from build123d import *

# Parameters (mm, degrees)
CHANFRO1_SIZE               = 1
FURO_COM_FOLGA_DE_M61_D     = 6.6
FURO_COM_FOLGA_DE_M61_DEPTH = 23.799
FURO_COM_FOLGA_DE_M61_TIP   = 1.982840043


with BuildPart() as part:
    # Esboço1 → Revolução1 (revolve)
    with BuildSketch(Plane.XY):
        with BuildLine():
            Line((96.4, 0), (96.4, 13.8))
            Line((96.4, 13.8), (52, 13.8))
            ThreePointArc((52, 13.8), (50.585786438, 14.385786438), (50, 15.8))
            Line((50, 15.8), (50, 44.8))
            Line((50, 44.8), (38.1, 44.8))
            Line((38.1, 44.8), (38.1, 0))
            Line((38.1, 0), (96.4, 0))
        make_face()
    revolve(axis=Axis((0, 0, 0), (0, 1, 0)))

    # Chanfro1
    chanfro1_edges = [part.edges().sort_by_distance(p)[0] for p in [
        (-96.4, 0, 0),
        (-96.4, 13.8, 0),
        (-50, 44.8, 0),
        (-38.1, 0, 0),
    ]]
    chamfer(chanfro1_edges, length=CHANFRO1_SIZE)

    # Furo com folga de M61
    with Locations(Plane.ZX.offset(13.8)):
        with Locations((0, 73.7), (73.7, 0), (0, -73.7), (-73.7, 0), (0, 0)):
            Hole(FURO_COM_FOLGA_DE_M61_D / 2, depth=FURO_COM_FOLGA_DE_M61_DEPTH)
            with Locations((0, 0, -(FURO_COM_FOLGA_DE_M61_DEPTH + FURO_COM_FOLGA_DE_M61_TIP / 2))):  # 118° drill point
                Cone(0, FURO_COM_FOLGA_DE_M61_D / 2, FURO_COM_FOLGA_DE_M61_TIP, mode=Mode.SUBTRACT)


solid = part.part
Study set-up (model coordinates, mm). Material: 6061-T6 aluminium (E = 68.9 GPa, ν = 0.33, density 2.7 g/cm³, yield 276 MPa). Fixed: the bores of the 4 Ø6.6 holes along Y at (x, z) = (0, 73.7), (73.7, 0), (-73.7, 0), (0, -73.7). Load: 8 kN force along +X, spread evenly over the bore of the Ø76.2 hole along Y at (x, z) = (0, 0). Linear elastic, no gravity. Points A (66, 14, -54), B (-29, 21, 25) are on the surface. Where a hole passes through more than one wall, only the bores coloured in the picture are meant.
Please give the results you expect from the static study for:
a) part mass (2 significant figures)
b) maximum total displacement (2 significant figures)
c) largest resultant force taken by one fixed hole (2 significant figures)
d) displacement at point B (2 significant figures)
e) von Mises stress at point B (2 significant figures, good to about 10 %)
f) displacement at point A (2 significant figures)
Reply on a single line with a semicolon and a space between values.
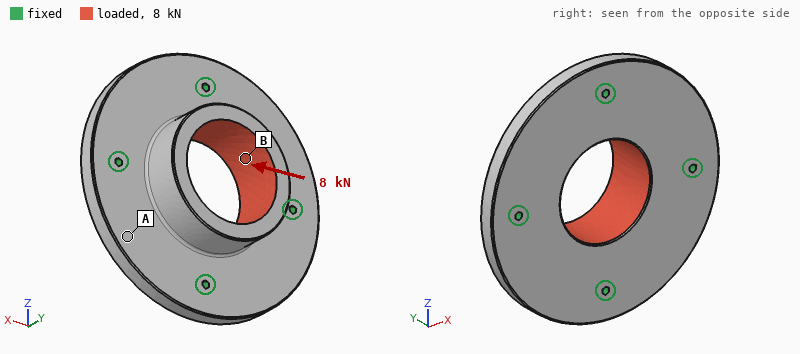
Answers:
1.2 kg; 9.2 µm; 2.4 kN; 4.7 µm; 3.3 MPa; 4.0 µm
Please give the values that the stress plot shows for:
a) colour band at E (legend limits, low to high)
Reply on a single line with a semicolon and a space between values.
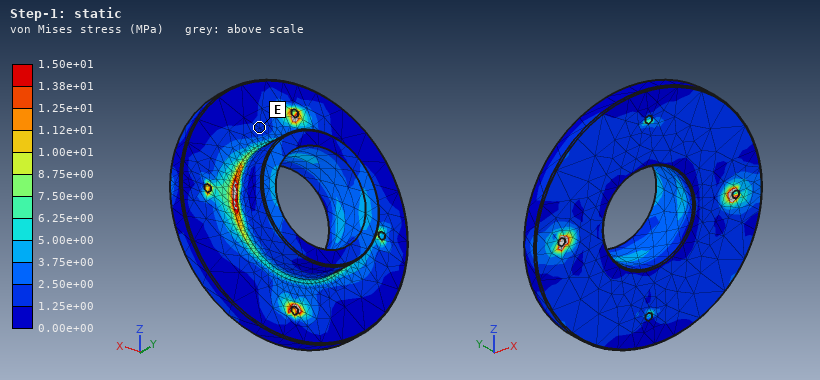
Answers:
1.25e+00 to 2.50e+00 MPa
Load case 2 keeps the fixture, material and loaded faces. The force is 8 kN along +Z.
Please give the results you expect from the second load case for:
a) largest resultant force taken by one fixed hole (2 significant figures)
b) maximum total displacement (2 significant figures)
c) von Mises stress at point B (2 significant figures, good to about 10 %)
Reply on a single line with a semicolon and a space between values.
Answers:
2.4 kN; 9.2 µm; 3.5 MPa
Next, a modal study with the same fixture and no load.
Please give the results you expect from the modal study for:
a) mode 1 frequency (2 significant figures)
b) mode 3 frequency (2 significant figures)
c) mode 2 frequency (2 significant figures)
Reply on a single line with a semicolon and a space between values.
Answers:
3700 Hz; 4100 Hz; 4100 Hz
